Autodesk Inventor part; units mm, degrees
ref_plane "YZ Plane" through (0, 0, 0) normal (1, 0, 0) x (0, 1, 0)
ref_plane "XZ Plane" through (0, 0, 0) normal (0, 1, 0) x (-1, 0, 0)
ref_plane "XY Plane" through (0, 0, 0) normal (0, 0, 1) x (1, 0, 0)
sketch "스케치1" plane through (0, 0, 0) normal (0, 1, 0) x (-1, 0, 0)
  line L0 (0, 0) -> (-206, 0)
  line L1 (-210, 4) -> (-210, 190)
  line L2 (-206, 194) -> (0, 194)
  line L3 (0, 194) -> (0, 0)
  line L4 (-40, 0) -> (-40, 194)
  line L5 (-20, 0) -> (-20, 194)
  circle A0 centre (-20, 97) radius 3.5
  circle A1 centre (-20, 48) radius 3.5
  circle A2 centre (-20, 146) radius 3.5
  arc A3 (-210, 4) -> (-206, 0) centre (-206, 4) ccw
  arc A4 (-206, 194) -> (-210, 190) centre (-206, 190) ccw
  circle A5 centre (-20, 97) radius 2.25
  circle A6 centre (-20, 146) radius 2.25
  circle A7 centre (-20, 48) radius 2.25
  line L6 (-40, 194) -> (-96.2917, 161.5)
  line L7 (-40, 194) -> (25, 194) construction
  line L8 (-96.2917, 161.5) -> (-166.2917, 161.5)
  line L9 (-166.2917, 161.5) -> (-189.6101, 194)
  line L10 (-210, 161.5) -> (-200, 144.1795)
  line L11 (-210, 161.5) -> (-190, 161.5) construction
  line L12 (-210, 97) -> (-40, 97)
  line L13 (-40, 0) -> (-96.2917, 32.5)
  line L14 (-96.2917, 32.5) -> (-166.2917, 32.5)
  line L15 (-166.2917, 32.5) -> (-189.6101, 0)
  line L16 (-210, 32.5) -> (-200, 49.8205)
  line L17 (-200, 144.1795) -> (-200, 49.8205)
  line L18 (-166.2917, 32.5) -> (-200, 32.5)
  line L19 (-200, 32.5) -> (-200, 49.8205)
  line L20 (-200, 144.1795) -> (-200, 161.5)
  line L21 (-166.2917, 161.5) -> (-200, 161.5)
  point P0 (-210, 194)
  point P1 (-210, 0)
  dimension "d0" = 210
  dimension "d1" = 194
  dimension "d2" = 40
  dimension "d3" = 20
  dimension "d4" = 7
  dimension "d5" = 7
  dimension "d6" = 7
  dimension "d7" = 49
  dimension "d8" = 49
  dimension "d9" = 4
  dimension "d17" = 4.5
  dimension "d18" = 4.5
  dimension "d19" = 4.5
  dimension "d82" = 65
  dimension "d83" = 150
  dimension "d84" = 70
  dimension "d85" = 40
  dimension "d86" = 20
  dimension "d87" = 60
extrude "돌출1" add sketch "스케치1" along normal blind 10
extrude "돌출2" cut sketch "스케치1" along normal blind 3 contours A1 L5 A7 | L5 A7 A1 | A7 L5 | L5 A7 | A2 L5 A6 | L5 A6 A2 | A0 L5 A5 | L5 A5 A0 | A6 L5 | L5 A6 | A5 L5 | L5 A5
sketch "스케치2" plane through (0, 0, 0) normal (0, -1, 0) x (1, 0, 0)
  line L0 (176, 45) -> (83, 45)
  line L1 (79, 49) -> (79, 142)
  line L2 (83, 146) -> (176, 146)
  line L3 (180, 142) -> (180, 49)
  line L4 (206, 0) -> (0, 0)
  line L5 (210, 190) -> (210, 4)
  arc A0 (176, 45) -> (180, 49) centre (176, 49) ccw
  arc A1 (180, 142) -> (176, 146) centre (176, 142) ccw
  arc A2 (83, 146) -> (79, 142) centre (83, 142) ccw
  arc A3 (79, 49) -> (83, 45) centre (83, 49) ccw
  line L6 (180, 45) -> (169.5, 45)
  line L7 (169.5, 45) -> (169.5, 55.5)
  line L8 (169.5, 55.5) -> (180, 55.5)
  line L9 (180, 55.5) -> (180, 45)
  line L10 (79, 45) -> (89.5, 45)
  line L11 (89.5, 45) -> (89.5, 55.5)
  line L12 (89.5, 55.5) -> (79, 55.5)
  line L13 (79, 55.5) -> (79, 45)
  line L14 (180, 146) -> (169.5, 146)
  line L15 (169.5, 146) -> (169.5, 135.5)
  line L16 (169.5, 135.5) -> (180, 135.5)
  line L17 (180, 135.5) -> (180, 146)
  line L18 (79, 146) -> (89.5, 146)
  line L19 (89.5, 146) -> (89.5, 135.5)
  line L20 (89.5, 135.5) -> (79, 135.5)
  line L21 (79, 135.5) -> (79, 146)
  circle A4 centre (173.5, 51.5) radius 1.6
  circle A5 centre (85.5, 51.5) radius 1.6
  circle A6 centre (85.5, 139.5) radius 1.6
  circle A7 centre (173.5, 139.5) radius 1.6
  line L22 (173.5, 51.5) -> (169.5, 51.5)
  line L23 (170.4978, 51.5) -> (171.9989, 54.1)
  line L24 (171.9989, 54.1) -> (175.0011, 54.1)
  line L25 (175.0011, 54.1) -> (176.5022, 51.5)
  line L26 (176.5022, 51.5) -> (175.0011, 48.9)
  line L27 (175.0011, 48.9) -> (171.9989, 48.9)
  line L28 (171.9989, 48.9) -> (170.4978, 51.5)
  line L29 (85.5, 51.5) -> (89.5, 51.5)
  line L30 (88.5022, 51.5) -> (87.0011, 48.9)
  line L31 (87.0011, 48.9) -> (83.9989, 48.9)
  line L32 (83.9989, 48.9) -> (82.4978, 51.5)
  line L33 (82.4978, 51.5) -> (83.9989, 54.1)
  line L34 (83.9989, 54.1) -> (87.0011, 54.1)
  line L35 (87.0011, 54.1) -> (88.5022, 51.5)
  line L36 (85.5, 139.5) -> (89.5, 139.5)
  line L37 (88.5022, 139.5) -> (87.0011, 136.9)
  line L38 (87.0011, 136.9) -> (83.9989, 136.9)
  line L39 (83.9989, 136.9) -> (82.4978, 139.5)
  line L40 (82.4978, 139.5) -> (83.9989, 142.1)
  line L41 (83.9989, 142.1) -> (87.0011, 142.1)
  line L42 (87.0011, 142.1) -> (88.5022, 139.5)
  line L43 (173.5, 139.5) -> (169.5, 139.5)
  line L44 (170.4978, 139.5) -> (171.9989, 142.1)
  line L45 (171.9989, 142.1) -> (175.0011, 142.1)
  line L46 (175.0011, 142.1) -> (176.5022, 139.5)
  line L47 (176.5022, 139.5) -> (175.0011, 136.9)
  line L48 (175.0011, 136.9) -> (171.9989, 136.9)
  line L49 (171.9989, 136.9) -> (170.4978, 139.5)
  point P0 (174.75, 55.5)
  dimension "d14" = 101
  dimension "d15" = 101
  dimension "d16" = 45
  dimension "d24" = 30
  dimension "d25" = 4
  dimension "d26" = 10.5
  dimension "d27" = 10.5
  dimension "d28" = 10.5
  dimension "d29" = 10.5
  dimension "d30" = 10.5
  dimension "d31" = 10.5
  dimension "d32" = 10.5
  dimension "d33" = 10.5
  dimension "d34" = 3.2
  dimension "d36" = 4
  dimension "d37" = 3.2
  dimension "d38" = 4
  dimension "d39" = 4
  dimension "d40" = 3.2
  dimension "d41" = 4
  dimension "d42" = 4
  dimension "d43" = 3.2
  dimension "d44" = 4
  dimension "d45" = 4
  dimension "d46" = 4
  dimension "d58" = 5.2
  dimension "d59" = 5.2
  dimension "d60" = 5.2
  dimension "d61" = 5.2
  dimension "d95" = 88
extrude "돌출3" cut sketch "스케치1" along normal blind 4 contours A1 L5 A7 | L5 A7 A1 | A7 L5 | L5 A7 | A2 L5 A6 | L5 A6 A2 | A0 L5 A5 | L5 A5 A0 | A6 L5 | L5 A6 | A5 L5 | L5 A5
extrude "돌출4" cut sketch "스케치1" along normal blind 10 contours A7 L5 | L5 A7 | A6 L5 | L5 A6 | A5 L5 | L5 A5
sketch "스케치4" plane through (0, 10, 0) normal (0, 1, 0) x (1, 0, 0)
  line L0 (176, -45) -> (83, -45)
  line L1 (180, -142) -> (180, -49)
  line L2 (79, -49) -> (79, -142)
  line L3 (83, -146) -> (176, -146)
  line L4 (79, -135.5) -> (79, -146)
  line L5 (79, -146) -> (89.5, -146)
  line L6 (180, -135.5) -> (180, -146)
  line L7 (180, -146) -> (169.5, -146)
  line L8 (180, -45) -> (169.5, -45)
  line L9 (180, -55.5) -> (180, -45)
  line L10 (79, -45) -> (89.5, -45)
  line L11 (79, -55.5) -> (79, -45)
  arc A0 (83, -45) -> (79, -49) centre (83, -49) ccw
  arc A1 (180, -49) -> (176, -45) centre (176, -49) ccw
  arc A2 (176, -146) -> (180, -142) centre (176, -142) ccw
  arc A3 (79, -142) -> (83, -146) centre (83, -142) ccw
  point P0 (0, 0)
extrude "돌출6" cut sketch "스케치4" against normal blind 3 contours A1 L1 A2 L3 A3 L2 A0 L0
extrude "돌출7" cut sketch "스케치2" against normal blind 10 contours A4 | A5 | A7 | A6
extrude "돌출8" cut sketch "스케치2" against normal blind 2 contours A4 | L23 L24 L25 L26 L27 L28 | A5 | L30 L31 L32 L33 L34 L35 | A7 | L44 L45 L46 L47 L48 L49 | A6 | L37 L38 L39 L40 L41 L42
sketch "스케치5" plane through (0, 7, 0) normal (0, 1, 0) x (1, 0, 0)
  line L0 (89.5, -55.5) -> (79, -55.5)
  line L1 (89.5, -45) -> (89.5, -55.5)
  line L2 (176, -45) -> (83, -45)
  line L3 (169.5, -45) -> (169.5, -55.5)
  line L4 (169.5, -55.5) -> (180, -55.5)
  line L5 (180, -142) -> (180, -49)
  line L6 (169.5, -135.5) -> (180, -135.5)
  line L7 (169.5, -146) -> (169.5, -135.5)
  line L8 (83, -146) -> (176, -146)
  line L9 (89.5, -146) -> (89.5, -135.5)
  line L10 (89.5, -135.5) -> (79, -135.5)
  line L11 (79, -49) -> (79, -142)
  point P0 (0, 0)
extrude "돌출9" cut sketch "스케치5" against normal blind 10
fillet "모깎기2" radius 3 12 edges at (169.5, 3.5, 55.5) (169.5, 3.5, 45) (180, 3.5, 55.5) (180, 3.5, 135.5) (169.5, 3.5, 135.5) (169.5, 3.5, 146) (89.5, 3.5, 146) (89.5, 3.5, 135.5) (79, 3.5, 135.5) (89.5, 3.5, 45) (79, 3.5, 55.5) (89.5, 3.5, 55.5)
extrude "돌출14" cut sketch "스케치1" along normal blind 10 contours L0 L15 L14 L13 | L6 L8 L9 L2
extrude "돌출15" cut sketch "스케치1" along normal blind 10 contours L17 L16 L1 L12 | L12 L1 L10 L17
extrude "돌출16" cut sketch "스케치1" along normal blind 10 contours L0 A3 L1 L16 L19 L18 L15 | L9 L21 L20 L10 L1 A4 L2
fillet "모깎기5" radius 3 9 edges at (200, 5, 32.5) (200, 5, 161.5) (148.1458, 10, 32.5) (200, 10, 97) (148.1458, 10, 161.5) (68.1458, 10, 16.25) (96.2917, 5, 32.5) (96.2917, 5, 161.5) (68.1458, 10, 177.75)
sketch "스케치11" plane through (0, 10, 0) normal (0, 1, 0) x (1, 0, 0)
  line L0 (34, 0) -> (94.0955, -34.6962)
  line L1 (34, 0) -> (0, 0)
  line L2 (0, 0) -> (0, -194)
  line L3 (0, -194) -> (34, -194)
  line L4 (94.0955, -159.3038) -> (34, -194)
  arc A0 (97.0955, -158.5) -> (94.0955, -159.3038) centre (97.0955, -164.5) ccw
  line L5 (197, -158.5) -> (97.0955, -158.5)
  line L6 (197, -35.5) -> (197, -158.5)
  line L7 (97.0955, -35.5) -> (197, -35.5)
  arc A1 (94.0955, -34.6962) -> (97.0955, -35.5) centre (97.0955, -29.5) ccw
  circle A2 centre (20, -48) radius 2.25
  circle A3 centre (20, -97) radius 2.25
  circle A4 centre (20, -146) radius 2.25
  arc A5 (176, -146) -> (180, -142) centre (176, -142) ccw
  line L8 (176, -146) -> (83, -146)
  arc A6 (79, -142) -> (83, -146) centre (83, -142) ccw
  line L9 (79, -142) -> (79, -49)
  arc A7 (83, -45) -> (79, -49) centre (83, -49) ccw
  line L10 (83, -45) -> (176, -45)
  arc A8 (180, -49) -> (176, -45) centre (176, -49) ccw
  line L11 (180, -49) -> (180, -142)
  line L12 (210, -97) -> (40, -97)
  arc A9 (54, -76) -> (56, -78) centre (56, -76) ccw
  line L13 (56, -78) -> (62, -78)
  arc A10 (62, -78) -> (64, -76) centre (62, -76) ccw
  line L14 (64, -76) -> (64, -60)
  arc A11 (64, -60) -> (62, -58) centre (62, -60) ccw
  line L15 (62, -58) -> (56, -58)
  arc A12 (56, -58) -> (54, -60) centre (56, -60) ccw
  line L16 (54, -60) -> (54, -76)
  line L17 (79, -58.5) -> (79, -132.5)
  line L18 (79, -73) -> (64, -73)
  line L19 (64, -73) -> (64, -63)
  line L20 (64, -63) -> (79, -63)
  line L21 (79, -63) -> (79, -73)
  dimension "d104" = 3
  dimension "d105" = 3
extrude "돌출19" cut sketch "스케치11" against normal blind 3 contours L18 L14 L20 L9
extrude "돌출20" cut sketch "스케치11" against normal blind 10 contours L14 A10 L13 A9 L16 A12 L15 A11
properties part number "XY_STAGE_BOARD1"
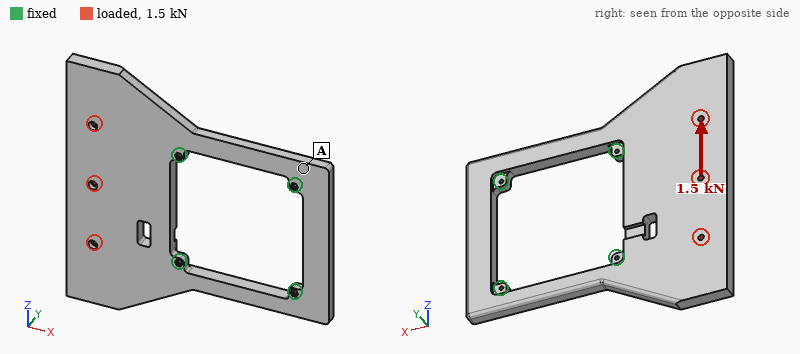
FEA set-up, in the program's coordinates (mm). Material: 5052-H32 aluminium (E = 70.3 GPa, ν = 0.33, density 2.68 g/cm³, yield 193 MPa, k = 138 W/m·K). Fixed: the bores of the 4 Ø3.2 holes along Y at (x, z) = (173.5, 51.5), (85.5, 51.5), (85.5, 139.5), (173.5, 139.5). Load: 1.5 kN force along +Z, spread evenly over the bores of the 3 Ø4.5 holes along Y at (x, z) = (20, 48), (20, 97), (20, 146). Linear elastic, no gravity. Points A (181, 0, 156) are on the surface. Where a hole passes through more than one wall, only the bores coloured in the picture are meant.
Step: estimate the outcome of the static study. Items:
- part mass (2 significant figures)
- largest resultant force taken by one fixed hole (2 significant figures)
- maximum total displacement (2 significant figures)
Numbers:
530 g
1.1 kN
24 µm
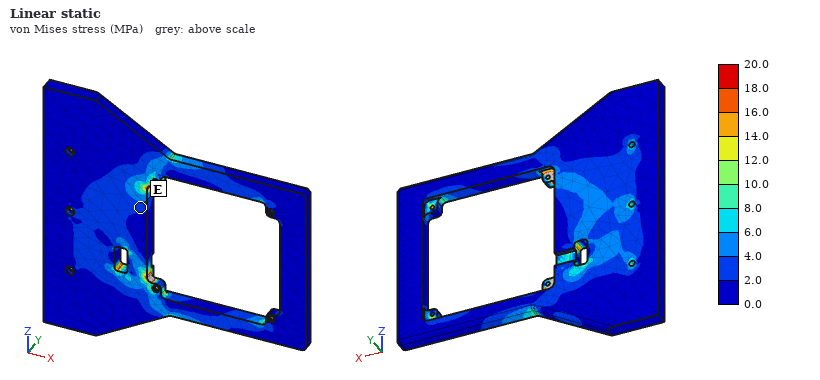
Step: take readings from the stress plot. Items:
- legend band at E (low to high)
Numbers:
2.0 to 4.0 MPa
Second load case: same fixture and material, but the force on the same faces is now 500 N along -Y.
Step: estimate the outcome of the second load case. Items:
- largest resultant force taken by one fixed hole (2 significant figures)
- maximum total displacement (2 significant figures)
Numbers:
410 N
0.37 mm
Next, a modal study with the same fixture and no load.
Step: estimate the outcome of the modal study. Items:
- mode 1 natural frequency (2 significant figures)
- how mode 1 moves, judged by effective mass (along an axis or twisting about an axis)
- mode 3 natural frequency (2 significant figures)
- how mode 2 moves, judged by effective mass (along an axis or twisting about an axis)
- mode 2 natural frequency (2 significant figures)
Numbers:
440 Hz
along Y
1600 Hz
twisting about X
860 Hz
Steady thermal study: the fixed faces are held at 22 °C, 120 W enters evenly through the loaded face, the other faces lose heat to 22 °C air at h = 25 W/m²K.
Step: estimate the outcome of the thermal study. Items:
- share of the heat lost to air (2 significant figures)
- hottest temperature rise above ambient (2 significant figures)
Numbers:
34 %
68 K
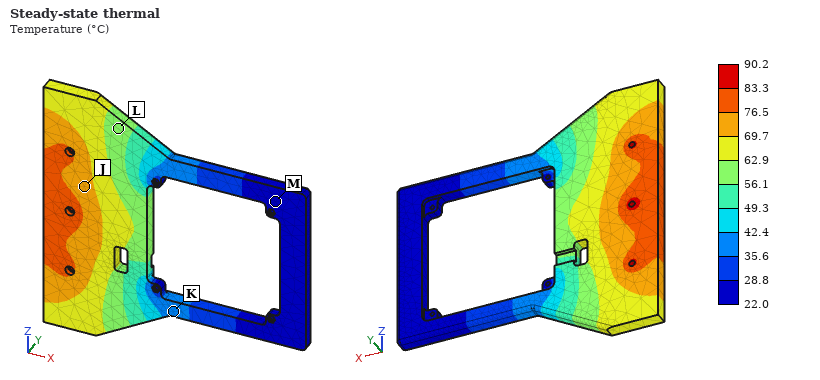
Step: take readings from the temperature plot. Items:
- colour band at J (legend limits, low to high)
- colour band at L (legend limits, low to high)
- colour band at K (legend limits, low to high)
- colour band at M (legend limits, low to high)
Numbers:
69.7 to 76.5 °C
56.1 to 62.9 °C
35.6 to 42.4 °C
22.0 to 28.8 °C
